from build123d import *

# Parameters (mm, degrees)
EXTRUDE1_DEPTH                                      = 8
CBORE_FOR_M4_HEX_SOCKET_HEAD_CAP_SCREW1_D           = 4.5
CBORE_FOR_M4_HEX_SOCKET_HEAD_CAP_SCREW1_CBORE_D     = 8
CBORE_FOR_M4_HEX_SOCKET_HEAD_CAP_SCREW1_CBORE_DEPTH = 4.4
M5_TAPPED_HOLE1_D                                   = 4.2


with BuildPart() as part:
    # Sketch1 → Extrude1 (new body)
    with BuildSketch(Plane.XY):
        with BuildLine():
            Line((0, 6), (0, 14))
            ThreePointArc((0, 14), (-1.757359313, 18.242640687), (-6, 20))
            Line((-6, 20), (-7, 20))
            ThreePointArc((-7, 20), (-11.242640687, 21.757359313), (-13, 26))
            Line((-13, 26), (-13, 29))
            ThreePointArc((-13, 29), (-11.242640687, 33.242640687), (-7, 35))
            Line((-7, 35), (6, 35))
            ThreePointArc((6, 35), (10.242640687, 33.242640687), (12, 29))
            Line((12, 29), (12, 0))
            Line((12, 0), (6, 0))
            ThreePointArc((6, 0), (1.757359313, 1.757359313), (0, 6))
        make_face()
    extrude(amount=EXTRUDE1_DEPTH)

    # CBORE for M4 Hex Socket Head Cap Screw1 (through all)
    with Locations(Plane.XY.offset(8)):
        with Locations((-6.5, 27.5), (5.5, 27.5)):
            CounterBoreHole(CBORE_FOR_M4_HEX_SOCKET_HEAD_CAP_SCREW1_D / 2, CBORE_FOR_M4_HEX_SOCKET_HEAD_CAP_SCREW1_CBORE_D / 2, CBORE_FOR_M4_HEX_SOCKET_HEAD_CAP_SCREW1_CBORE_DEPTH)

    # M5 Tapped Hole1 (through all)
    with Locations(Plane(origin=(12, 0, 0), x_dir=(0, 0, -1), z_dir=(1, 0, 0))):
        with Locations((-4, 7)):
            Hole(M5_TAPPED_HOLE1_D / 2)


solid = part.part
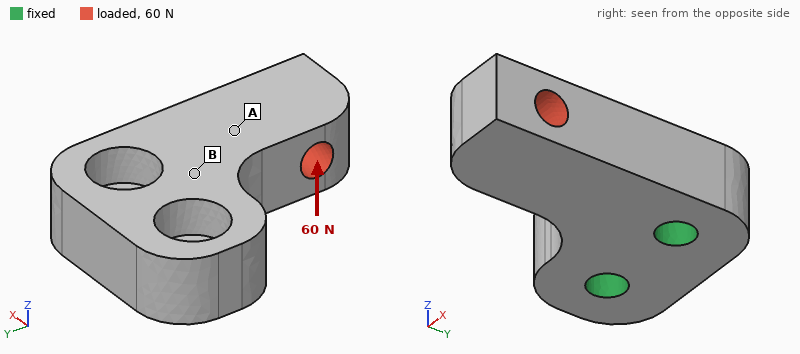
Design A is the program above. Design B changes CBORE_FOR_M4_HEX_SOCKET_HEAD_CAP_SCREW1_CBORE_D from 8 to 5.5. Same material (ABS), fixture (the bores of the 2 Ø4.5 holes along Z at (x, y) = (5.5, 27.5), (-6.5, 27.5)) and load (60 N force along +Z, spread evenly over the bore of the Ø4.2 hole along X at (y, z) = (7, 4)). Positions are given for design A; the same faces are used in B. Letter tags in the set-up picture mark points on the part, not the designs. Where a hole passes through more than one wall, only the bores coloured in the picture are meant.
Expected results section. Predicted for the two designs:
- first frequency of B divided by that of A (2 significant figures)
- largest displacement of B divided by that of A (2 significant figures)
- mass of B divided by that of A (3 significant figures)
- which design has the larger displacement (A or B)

1.1
0.85
1.06
A
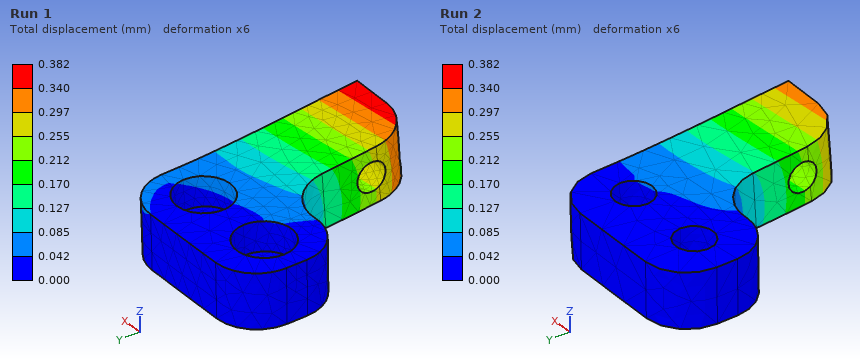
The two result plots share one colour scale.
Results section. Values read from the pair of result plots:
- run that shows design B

Run 2
